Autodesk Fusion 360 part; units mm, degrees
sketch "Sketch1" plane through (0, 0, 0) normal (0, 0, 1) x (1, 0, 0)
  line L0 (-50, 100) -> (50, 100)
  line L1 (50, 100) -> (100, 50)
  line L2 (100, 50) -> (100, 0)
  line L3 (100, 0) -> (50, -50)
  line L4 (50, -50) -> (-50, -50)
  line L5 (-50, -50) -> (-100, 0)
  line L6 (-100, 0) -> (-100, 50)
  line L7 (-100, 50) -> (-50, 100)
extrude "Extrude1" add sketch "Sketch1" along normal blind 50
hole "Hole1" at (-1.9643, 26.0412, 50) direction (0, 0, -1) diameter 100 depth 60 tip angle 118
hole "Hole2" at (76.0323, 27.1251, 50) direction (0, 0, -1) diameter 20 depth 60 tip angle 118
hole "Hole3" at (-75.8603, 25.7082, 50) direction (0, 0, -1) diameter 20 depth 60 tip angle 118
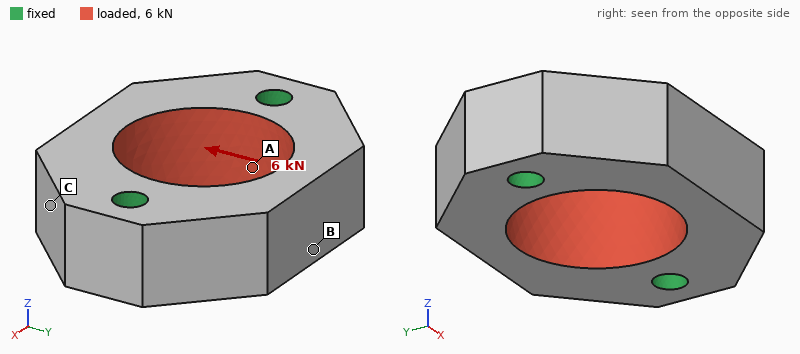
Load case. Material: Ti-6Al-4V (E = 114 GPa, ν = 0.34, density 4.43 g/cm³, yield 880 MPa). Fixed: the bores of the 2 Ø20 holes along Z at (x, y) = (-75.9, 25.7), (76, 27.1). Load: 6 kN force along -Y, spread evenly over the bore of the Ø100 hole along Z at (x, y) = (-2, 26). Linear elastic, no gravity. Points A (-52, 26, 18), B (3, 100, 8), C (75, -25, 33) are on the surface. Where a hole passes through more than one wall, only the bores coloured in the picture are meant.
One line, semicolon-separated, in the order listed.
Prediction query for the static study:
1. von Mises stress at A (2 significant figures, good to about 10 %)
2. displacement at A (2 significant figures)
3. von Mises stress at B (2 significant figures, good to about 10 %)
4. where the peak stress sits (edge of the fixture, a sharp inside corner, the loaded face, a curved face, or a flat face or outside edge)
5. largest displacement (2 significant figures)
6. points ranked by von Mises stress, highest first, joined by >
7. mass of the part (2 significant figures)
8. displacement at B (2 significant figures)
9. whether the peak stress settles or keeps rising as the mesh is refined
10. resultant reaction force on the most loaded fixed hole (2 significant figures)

0.63 MPa; 0.29 µm; 1.7 MPa; edge of the fixture; 1.3 µm; B > A > C; 3.7 kg; 1.1 µm; keeps rising; 3.0 kN
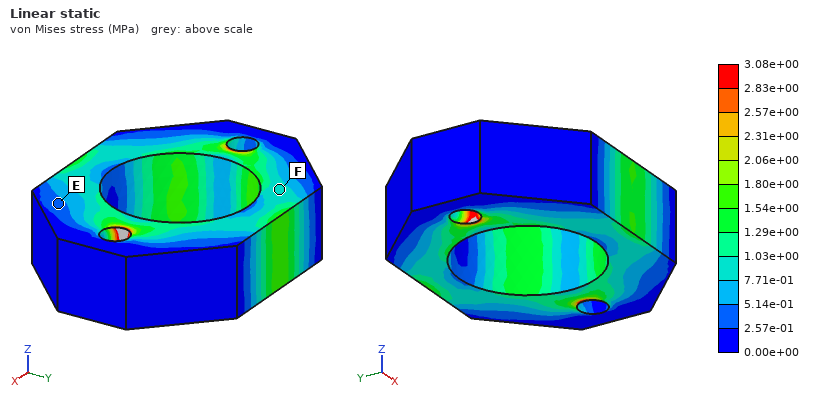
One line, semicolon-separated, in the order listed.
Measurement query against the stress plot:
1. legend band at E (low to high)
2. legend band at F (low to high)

2.57e-01 to 5.14e-01 MPa; 7.71e-01 to 1.03e+00 MPa
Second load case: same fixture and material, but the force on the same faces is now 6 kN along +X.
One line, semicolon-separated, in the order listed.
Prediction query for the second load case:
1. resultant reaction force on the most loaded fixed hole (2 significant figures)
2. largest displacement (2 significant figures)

3.1 kN; 1.1 µm
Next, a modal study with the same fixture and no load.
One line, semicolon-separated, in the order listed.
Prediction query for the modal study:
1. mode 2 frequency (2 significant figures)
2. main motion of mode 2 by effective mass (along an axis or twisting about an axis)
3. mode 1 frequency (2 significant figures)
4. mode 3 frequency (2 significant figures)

4700 Hz; along Z; 4300 Hz; 5900 Hz
